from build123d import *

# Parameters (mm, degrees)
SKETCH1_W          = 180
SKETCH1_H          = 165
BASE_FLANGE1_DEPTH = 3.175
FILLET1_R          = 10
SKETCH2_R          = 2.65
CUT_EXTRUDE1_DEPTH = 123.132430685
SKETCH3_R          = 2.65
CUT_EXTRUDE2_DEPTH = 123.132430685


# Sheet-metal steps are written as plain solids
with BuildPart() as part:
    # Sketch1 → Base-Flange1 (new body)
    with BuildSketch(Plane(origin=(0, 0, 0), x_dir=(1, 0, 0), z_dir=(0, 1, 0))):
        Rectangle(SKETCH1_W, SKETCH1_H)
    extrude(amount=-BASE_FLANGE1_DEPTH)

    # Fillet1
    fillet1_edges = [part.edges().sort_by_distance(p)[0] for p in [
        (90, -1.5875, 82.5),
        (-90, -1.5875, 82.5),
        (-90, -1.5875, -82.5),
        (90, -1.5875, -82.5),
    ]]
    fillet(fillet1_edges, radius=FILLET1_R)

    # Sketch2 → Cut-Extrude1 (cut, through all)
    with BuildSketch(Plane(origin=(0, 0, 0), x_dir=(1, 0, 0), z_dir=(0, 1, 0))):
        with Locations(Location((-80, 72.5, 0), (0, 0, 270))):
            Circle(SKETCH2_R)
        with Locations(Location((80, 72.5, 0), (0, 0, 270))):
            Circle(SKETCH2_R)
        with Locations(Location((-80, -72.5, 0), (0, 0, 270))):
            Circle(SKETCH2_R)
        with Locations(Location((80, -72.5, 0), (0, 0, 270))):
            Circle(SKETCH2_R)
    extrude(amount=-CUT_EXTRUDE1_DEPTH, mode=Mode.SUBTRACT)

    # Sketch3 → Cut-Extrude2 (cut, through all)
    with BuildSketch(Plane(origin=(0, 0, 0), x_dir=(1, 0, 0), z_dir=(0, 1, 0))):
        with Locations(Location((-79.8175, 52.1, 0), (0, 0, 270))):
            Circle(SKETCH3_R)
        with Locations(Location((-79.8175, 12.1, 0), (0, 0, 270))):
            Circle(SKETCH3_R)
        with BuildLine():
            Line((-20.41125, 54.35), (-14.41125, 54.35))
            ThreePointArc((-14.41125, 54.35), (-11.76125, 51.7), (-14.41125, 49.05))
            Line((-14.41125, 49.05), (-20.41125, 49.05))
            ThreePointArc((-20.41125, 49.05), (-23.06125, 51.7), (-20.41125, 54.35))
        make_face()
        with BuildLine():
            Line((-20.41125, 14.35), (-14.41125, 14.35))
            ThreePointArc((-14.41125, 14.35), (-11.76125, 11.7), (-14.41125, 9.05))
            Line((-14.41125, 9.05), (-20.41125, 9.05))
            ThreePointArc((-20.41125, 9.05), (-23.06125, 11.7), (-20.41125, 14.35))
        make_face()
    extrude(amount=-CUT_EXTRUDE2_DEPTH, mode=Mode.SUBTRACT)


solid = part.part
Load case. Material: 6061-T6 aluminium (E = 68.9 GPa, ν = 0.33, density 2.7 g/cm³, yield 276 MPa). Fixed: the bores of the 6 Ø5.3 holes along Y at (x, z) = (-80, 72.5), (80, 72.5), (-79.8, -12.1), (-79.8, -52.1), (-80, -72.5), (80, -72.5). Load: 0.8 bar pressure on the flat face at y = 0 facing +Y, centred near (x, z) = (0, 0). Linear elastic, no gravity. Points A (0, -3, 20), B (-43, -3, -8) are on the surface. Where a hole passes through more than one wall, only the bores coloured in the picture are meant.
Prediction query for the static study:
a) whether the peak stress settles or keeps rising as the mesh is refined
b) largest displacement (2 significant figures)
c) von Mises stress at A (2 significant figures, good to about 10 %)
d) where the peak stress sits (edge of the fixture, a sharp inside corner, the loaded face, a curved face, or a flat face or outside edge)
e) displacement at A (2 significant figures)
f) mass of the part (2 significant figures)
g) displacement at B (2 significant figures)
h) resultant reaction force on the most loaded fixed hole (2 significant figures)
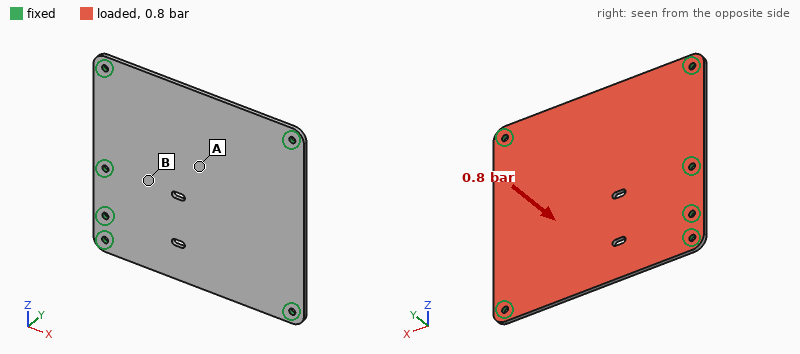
keeps rising
1.3 mm
55 MPa
edge of the fixture
1.2 mm
250 g
0.58 mm
560 N
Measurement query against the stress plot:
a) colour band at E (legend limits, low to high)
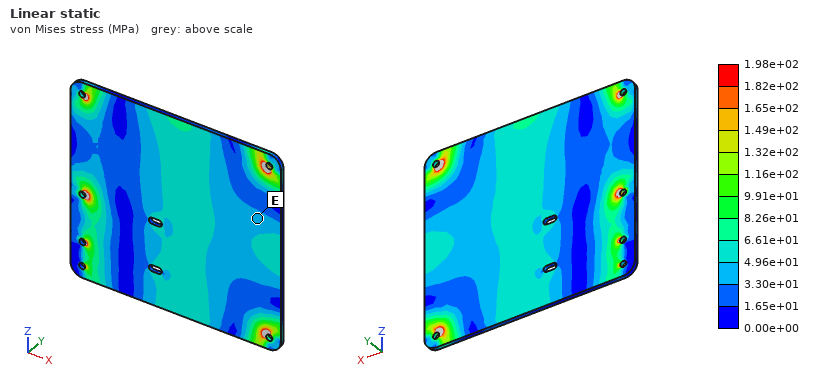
3.30e+01 to 4.96e+01 MPa
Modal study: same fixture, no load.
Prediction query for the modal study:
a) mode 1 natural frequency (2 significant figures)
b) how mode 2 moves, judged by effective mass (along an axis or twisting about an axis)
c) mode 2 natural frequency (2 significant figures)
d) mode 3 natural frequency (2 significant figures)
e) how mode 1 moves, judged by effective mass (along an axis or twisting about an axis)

510 Hz
twisting about X
750 Hz
860 Hz
along Y
